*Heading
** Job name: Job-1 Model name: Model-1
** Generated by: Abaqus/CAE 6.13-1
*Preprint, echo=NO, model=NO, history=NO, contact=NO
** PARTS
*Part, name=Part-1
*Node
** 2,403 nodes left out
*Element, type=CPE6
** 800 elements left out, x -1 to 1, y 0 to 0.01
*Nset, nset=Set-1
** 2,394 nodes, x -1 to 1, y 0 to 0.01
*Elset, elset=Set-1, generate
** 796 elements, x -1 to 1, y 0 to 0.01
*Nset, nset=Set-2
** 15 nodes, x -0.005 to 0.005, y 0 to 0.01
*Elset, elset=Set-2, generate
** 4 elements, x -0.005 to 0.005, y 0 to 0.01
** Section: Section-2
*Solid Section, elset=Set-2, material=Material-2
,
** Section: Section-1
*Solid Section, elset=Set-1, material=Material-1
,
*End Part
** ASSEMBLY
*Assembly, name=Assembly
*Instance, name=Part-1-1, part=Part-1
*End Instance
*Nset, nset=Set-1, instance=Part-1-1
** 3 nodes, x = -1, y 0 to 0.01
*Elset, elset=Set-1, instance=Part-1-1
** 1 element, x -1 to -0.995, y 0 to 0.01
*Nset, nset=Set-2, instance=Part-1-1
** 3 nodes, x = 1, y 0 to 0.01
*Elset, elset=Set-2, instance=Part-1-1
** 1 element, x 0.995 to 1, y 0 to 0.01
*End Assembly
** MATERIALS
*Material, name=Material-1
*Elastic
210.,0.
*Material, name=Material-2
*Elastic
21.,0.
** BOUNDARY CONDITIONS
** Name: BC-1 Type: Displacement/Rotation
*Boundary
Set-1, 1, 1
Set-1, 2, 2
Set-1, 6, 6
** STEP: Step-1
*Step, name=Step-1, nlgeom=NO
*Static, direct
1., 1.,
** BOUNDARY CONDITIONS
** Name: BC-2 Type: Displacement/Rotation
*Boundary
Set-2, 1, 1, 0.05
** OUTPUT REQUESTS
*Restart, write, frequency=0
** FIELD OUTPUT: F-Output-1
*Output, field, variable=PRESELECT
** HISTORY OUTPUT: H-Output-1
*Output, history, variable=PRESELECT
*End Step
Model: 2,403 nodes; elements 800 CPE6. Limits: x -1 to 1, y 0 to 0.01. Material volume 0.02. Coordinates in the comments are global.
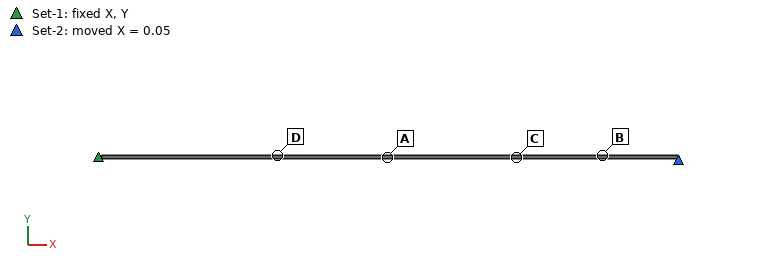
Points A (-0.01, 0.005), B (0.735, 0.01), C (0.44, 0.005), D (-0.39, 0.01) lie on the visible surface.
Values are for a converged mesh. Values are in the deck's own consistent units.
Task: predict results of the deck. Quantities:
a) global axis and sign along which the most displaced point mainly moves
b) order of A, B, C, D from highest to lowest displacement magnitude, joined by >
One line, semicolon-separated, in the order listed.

+X; B > C > A > D
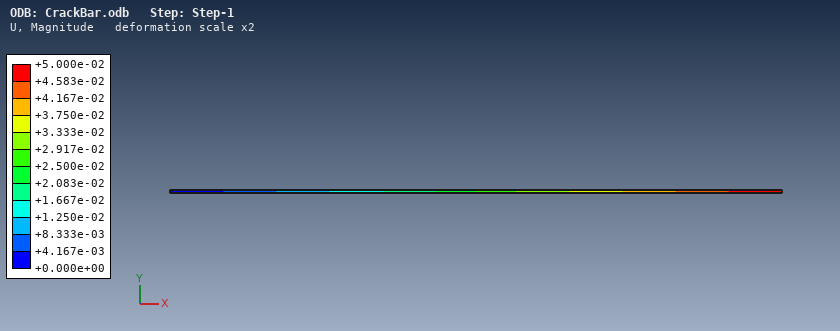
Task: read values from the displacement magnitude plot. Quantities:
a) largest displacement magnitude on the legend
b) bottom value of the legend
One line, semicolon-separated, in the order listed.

+5.000e-02; +0.000e+00
